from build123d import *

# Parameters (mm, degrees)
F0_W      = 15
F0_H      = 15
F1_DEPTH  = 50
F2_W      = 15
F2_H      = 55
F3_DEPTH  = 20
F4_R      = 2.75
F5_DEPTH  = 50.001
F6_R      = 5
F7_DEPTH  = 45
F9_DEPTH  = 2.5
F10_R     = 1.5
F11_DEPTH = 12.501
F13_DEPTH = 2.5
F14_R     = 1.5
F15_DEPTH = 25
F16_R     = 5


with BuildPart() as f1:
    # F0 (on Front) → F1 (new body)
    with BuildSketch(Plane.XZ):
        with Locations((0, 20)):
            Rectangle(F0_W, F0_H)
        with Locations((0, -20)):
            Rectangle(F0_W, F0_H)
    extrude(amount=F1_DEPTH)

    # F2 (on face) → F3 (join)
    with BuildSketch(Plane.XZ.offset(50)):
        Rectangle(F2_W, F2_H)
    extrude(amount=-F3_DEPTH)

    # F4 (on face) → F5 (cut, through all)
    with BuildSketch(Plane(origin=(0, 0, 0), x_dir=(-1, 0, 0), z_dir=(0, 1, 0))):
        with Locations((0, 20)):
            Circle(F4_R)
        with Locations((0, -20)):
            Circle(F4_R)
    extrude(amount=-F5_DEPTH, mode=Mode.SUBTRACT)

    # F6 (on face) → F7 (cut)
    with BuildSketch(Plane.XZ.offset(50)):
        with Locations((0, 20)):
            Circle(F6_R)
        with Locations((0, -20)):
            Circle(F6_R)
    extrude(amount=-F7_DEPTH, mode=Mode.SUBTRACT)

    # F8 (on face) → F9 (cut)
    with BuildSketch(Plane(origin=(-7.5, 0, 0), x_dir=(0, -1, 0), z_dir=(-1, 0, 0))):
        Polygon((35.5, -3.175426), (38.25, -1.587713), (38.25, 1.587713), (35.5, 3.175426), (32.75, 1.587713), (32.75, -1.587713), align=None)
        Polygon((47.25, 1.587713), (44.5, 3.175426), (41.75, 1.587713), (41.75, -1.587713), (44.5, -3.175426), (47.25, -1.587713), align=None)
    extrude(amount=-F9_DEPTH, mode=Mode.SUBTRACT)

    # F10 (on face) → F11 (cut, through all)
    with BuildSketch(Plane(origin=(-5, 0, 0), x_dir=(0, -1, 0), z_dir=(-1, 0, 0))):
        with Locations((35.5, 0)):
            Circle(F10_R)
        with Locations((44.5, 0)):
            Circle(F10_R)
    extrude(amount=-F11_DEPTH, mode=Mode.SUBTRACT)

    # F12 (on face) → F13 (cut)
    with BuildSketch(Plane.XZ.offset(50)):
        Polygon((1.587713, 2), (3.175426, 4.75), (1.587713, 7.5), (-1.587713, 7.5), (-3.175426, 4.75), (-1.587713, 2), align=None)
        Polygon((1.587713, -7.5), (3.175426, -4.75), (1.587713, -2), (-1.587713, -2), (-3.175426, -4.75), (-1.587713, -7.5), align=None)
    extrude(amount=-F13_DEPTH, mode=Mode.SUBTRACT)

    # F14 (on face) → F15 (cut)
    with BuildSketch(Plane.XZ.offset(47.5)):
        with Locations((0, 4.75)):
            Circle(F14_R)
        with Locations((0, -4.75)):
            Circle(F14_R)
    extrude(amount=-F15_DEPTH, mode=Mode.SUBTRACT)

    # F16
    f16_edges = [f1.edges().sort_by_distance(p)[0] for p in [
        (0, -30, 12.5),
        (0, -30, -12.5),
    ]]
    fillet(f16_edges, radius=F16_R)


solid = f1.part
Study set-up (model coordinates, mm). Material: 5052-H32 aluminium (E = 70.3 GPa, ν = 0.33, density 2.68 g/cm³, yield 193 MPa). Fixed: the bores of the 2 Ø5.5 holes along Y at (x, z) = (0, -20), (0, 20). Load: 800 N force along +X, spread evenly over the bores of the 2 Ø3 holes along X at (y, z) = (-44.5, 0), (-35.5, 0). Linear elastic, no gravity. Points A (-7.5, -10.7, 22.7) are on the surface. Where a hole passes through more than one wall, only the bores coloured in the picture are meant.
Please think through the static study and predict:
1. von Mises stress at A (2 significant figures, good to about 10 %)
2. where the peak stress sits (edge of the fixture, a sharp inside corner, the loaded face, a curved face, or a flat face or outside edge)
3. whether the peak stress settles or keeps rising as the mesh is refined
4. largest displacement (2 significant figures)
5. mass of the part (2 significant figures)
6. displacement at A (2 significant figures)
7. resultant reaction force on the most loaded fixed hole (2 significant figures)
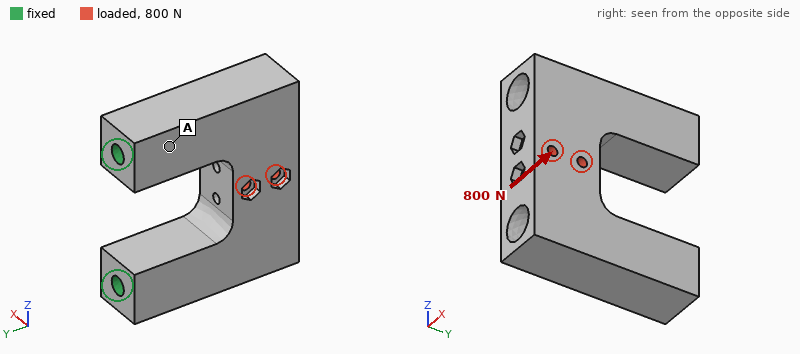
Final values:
24 MPa
edge of the fixture
keeps rising
0.11 mm
59 g
0.019 mm
400 N
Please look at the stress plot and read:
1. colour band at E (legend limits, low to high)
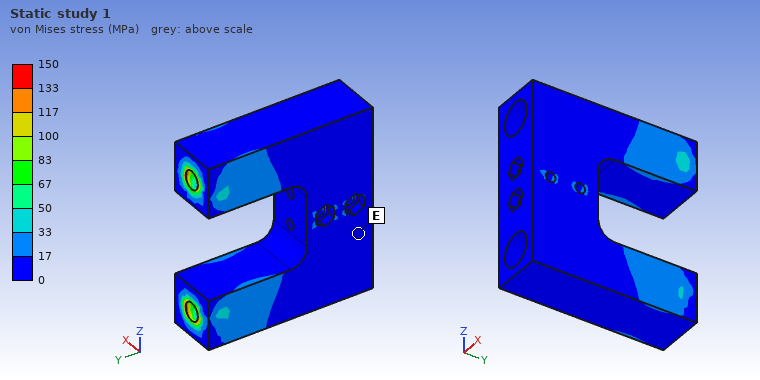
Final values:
0 to 17 MPa
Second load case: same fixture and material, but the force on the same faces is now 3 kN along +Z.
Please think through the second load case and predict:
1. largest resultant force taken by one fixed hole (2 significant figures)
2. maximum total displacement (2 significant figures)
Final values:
2.5 kN
81 µm
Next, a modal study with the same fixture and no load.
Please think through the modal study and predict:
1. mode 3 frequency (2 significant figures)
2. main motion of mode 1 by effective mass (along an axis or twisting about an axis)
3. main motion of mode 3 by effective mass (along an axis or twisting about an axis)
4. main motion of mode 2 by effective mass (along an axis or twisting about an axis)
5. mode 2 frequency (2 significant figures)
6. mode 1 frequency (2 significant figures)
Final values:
6300 Hz
along X
twisting about Y
along Z
5100 Hz
2500 Hz
